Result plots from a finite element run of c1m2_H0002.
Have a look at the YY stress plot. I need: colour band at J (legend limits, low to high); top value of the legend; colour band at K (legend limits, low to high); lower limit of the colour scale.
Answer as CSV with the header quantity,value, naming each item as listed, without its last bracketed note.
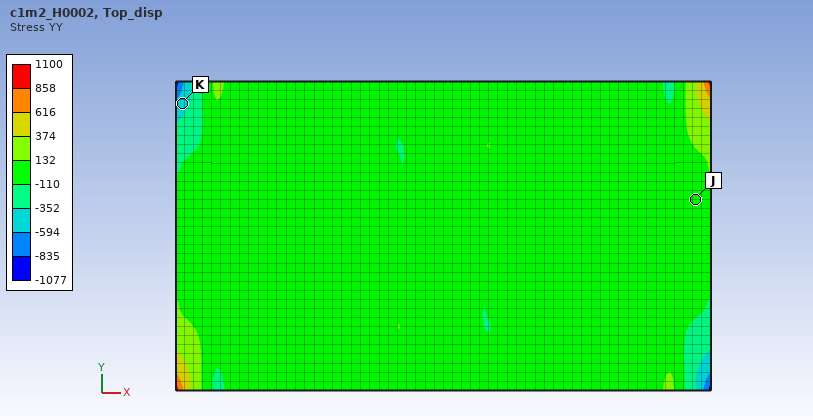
quantity,value
colour band at J,-110 to 132
top value of the legend,1100
colour band at K,-594 to -352
lower limit of the colour scale,-1077
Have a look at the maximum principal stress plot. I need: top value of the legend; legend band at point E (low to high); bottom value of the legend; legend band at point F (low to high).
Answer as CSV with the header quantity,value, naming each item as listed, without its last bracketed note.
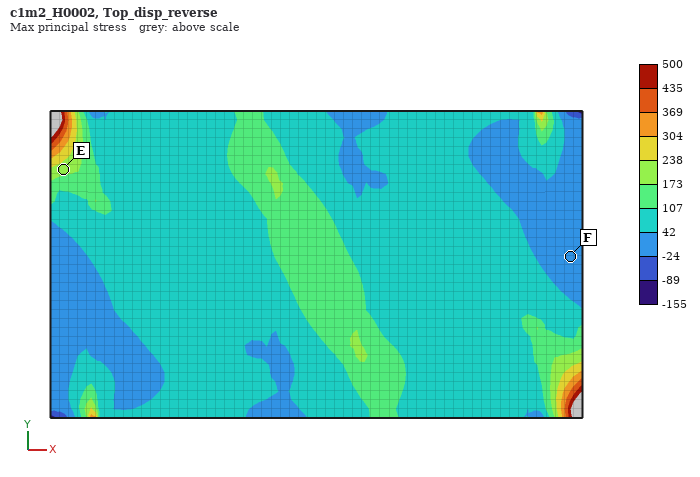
quantity,value
top value of the legend,500
legend band at point E,173 to 238
bottom value of the legend,-155
legend band at point F,-24 to 42
